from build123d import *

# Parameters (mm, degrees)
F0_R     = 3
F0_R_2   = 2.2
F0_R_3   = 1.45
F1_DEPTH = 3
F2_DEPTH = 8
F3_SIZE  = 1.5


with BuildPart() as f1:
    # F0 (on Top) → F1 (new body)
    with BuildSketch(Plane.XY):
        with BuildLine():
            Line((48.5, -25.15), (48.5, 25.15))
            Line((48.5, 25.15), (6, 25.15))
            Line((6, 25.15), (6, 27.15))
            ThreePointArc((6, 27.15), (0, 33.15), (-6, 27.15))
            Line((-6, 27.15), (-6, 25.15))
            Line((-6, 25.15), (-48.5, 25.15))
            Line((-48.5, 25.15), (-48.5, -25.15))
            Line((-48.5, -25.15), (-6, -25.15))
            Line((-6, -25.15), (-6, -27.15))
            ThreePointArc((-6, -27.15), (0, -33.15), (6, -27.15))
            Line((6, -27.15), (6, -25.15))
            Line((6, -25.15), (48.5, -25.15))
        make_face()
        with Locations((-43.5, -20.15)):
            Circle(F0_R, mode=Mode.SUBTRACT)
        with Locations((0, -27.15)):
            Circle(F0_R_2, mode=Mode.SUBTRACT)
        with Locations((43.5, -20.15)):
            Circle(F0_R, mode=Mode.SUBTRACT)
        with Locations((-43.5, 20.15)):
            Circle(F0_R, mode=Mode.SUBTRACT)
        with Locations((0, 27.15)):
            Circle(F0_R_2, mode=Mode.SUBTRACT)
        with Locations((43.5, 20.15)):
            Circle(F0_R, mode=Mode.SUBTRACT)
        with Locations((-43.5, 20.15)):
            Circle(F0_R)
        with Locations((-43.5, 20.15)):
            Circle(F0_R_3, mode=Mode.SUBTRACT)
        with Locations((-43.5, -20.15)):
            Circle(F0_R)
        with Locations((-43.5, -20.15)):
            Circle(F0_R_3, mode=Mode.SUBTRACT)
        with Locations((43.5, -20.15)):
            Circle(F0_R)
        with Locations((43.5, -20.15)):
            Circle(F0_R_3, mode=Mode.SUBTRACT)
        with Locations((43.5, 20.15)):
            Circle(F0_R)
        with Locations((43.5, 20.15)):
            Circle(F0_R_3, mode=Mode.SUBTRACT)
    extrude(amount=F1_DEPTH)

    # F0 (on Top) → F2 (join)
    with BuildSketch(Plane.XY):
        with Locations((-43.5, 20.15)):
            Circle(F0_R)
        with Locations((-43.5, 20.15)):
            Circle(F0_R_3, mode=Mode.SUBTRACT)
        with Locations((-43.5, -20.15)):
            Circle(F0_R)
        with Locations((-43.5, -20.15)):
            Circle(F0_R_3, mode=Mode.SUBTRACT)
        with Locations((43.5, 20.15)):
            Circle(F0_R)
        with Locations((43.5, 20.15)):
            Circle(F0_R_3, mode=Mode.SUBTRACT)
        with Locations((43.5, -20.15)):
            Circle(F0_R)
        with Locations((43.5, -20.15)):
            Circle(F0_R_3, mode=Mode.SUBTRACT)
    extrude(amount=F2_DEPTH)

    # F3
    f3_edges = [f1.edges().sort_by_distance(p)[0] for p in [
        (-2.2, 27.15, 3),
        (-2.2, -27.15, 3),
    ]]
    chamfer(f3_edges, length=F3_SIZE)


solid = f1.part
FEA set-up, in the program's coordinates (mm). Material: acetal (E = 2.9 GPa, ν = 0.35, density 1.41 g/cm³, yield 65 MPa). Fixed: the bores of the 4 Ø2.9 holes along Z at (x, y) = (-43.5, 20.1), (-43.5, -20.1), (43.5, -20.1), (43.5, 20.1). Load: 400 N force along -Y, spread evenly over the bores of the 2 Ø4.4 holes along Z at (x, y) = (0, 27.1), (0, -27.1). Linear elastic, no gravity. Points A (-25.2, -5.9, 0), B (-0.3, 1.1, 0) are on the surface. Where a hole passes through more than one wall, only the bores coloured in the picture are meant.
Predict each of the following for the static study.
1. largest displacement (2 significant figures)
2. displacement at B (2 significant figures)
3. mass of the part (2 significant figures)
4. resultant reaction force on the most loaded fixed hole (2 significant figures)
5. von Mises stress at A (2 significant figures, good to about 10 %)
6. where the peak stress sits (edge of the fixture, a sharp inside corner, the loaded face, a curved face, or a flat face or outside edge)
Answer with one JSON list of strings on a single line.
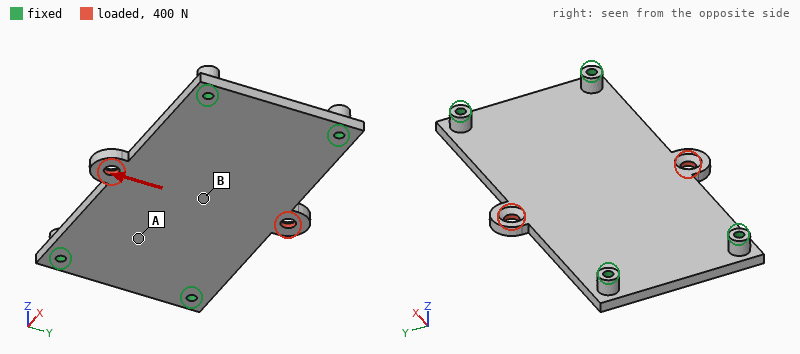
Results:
["0.40 mm", "0.075 mm", "22 g", "130 N", "4.3 MPa", "the loaded face"]
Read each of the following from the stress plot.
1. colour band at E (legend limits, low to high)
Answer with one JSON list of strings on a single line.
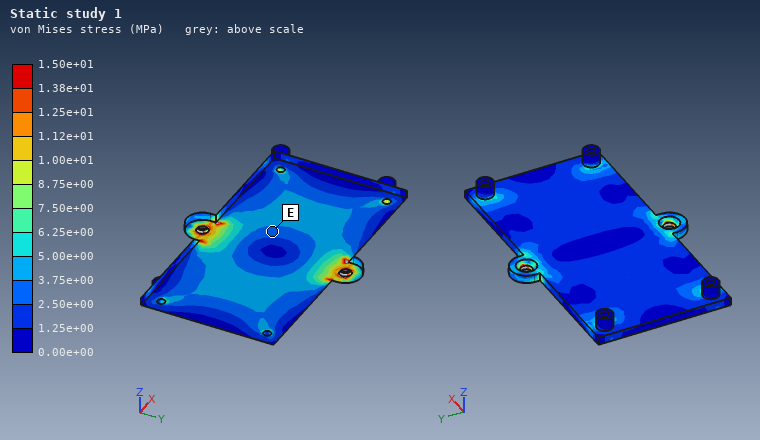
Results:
["2.50e+00 to 3.75e+00 MPa"]
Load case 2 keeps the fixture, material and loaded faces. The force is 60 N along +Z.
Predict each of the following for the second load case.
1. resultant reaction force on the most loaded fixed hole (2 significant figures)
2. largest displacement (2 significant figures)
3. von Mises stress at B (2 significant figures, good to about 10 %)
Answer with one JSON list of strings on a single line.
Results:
["16 N", "1.2 mm", "6.9 MPa"]
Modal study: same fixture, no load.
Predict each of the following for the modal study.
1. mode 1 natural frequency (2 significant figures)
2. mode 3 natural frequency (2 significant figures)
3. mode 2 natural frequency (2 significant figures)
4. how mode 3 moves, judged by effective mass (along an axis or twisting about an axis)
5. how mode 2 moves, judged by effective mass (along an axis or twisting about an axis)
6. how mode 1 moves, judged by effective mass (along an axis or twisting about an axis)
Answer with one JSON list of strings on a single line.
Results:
["520 Hz", "1500 Hz", "800 Hz", "twisting about Y", "twisting about X", "along Z"]
